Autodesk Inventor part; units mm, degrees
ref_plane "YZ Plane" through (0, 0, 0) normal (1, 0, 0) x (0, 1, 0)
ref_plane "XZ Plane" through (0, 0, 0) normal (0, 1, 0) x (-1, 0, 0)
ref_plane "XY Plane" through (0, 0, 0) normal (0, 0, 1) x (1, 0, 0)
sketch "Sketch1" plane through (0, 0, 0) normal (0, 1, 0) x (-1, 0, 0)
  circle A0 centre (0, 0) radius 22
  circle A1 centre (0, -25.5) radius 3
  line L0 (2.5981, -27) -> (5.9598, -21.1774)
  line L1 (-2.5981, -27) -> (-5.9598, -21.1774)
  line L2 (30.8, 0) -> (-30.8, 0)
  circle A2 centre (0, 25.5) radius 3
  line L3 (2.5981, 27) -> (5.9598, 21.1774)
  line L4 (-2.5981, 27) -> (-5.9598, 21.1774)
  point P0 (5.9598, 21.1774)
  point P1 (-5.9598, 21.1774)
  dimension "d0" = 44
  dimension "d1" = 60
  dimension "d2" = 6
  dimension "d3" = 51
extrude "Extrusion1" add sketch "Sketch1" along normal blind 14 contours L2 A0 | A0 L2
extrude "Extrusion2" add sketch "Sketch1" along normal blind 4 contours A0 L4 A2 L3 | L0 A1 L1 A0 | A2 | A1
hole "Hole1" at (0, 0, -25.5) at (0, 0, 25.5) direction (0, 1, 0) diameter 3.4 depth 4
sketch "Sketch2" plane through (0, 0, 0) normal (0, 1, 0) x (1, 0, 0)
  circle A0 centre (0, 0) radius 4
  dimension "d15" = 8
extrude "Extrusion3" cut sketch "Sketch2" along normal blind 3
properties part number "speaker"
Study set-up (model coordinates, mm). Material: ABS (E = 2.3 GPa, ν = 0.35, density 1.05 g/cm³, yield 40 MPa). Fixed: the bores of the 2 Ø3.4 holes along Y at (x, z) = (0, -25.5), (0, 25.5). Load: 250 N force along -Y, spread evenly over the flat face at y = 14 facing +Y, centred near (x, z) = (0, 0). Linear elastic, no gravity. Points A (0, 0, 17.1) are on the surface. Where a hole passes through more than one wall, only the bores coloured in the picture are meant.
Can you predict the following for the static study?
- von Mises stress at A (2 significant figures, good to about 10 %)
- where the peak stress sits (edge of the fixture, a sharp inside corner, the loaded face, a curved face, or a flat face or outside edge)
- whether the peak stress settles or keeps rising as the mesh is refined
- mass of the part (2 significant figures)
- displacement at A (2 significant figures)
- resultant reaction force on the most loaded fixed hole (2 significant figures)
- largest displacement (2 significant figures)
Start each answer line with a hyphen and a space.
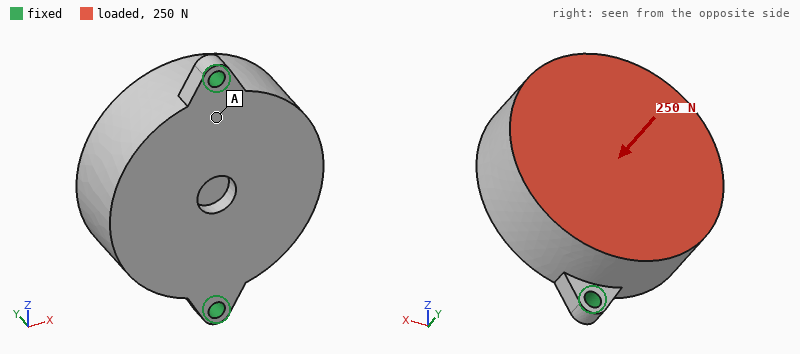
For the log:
- 1.6 MPa
- edge of the fixture
- keeps rising
- 23 g
- 37 µm
- 150 N
- 59 µm
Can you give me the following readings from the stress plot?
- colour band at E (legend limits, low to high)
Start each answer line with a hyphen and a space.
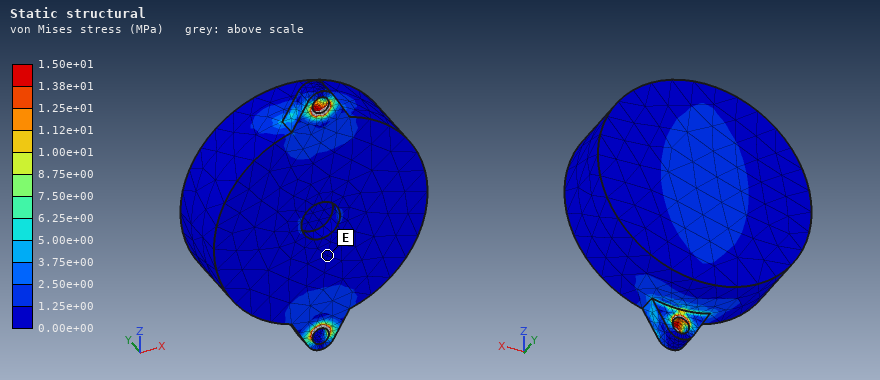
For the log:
- 0.00e+00 to 1.25e+00 MPa
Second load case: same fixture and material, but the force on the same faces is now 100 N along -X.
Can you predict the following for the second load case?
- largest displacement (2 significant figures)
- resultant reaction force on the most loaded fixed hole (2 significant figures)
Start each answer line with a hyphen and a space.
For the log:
- 0.43 mm
- 50 N
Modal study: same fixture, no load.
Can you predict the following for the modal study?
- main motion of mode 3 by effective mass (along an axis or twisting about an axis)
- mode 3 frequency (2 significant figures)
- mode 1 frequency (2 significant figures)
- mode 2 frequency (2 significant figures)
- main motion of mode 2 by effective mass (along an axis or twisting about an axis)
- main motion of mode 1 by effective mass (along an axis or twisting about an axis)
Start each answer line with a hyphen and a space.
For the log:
- along X
- 3500 Hz
- 700 Hz
- 2400 Hz
- along Y
- along X
